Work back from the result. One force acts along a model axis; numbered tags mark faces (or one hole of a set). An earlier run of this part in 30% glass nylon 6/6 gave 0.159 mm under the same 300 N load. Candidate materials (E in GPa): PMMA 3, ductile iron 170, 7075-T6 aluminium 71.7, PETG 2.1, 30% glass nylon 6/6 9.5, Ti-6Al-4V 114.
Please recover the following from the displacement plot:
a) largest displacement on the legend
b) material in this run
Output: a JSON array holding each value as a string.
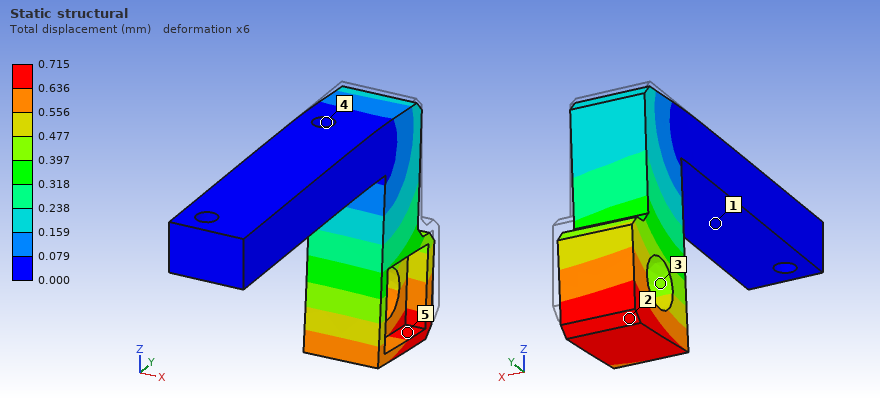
["0.715 mm", "PETG"]
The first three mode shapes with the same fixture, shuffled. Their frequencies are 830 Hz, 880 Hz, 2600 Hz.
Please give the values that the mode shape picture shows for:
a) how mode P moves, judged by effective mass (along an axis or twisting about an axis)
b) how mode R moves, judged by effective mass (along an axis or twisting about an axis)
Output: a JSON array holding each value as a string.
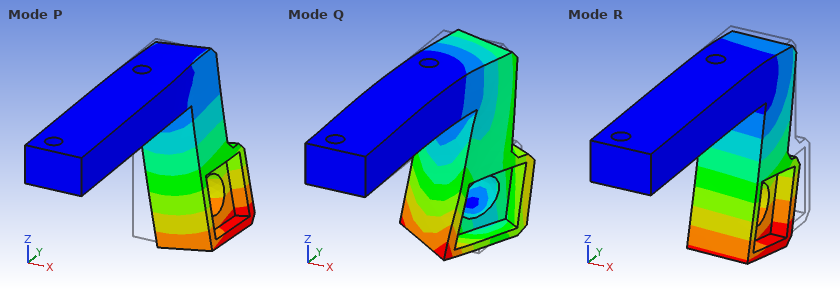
["along X", "along Y"]
